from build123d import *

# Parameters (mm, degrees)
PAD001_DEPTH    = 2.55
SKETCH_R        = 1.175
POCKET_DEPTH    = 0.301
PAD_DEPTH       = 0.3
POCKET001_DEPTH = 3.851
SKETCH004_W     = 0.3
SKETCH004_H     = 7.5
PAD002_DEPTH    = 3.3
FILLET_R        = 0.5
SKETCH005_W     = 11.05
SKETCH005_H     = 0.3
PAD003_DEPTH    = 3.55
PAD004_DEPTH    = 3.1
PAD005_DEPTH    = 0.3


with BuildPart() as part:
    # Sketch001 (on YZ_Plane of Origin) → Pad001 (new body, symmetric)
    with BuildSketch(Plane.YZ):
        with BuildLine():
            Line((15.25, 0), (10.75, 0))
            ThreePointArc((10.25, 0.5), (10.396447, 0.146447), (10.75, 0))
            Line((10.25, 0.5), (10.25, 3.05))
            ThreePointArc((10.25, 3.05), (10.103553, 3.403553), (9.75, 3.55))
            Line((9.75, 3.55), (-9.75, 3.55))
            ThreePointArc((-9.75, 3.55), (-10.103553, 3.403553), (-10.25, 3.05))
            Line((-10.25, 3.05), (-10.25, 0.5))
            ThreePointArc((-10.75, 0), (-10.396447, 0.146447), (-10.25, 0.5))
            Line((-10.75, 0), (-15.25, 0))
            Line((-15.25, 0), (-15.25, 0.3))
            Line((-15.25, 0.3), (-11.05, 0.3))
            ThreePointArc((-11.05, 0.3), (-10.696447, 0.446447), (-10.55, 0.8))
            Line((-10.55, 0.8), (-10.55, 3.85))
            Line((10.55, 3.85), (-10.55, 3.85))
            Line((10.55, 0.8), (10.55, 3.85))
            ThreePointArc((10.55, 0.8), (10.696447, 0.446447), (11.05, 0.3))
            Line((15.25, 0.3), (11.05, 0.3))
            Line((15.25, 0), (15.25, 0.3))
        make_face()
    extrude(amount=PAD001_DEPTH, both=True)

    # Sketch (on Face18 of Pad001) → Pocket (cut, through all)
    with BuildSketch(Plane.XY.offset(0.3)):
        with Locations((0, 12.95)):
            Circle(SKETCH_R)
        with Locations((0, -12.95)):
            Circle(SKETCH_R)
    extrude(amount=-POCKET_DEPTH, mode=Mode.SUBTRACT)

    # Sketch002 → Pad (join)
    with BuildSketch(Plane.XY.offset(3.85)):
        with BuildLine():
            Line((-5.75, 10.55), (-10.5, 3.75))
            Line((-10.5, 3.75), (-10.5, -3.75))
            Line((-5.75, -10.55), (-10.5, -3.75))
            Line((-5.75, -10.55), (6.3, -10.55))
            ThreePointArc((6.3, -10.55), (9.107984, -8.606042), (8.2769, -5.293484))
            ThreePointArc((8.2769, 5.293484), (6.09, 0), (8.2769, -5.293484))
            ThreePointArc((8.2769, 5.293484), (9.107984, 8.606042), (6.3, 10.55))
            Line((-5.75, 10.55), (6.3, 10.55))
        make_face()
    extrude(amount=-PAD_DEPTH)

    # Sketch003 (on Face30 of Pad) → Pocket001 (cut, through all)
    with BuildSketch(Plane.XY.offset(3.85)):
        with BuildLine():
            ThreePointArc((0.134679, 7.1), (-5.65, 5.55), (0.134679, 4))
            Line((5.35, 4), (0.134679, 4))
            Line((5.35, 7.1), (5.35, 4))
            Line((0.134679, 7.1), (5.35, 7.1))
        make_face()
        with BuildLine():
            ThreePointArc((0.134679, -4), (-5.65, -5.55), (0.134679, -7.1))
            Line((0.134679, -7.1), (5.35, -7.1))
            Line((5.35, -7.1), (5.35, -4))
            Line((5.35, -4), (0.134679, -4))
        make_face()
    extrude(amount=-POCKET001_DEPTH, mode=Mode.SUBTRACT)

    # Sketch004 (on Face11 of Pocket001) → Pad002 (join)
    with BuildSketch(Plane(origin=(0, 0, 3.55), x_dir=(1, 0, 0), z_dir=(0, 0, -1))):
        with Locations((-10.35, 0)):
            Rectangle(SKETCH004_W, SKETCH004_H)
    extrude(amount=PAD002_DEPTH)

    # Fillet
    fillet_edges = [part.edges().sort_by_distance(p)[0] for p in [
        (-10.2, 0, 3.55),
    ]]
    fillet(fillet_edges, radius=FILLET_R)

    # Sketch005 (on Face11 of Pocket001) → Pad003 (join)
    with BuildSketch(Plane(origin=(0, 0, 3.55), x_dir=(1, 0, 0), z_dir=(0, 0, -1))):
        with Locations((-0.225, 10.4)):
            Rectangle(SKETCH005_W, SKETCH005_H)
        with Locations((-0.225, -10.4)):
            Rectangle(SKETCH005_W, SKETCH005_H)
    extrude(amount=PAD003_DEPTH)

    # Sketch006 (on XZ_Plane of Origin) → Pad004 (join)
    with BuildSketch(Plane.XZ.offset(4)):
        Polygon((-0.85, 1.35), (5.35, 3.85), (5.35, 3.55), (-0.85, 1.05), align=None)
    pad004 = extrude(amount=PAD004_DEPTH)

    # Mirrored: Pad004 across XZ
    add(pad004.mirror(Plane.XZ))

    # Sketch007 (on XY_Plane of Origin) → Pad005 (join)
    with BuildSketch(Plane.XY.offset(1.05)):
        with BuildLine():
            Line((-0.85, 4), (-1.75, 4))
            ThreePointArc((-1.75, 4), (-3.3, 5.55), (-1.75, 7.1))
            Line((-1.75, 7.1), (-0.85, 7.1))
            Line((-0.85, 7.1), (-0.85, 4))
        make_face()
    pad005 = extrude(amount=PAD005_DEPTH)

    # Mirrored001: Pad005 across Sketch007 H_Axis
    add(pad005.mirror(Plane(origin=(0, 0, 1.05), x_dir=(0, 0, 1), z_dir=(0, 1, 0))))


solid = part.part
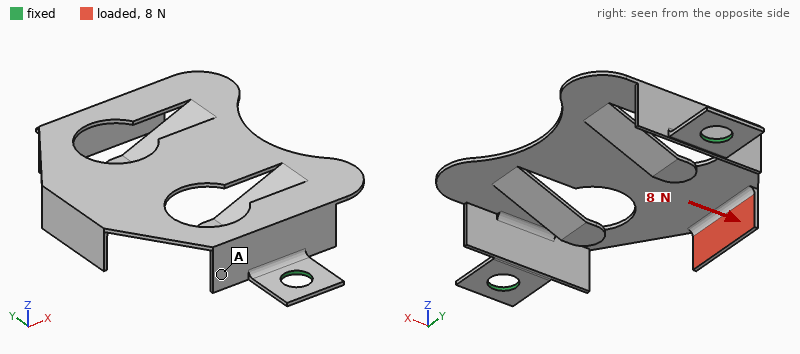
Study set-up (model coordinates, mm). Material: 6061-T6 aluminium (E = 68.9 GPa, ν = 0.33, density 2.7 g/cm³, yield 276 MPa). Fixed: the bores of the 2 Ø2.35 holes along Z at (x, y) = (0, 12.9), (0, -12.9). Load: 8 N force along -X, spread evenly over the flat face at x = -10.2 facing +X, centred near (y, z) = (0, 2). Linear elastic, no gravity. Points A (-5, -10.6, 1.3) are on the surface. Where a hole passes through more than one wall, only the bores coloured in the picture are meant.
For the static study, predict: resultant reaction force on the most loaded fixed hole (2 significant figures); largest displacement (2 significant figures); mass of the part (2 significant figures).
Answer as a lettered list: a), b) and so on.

a) 4.0 N
b) 0.38 mm
c) 0.37 g
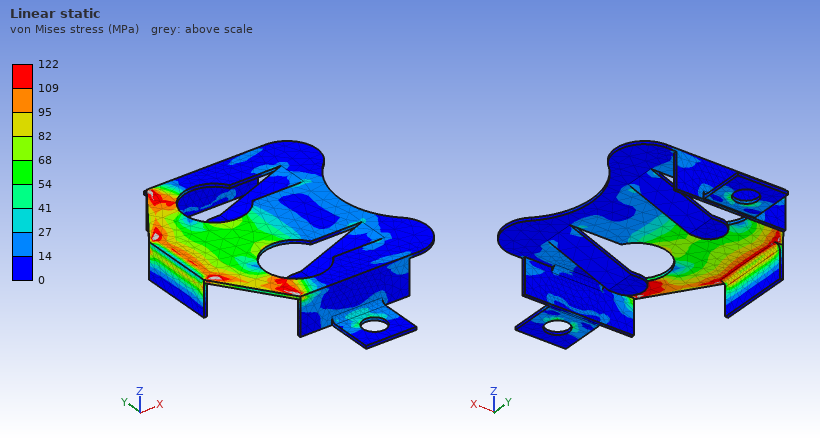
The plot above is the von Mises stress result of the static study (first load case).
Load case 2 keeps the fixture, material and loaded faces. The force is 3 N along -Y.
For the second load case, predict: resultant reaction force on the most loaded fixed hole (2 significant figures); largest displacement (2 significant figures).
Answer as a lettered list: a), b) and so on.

a) 2.2 N
b) 0.10 mm
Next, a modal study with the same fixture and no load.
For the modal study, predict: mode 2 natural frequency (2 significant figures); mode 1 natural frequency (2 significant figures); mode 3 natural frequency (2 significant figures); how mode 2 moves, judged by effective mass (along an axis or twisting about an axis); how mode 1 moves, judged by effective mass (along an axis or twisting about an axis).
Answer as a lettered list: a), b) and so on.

a) 2300 Hz
b) 1800 Hz
c) 2500 Hz
d) along Z
e) along Z
